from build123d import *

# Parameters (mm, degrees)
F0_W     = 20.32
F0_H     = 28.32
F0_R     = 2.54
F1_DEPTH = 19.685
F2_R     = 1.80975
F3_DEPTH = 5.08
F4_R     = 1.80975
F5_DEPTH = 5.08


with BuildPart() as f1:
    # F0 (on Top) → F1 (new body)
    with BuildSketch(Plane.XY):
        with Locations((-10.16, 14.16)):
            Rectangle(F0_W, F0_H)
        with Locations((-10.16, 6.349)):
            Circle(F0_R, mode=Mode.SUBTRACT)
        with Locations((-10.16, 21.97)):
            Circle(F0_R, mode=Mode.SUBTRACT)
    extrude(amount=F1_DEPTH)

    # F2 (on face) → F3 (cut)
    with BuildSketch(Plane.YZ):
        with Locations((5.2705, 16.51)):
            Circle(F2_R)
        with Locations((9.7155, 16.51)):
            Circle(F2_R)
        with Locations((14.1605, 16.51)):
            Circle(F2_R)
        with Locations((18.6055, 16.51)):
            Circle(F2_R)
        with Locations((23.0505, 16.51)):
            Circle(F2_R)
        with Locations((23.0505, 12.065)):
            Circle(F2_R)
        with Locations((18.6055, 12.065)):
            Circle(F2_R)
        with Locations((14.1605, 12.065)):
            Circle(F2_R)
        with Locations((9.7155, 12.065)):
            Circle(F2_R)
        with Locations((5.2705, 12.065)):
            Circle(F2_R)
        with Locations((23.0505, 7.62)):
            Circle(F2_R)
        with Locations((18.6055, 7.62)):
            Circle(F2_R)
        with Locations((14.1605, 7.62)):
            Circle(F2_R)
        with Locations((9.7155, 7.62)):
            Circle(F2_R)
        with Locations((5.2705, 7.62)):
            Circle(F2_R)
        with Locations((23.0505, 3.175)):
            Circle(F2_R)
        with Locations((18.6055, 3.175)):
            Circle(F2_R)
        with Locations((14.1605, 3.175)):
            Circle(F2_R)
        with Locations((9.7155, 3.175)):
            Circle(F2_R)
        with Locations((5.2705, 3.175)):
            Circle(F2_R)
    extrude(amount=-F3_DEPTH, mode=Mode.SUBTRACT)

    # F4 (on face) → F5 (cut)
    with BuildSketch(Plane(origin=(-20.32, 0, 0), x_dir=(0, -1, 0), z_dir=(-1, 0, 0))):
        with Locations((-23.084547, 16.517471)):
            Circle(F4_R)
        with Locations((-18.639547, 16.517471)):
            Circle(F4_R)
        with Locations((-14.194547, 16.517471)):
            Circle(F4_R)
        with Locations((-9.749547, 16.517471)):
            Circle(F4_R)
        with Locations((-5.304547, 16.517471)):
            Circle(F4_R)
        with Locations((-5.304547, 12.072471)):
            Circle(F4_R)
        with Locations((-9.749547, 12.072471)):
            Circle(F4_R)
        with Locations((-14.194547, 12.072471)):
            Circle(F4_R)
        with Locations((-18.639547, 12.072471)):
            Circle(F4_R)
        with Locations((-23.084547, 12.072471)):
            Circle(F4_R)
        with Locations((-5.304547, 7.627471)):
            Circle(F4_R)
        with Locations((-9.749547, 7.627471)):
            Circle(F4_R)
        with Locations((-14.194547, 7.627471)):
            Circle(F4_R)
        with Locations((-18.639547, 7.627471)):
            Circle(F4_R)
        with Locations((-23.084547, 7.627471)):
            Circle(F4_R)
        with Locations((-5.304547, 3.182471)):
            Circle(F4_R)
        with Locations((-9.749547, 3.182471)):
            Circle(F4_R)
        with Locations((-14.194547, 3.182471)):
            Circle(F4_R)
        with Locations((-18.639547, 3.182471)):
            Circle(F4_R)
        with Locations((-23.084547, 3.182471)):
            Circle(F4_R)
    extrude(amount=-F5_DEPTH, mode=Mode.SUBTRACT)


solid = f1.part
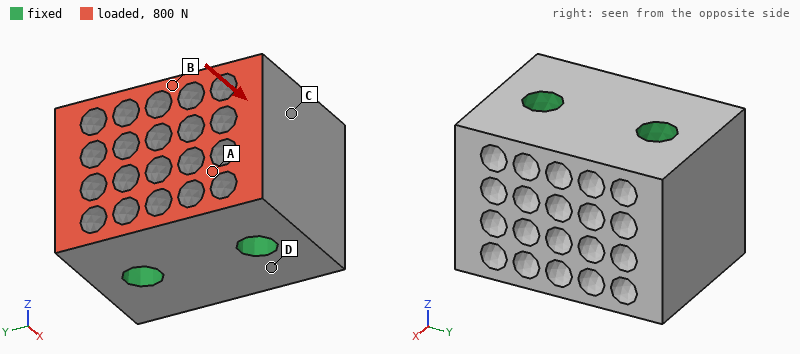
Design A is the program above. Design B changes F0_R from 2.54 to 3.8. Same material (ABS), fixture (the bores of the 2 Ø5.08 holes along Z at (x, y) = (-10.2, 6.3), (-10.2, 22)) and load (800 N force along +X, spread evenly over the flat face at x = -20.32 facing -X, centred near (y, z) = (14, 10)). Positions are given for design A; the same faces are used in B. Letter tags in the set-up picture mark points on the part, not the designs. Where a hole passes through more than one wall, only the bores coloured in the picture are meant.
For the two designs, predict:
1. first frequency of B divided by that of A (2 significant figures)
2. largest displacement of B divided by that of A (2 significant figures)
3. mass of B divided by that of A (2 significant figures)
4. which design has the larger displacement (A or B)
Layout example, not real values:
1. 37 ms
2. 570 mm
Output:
1. 1.3
2. 0.85
3. 0.88
4. A
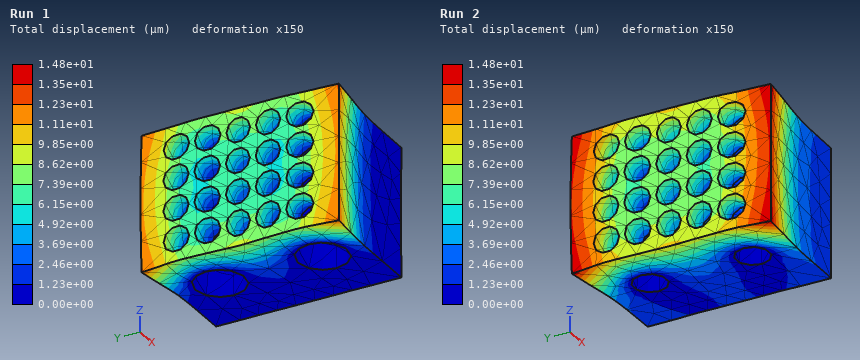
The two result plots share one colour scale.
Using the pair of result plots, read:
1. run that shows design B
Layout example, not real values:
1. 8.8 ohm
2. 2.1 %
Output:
1. Run 1
